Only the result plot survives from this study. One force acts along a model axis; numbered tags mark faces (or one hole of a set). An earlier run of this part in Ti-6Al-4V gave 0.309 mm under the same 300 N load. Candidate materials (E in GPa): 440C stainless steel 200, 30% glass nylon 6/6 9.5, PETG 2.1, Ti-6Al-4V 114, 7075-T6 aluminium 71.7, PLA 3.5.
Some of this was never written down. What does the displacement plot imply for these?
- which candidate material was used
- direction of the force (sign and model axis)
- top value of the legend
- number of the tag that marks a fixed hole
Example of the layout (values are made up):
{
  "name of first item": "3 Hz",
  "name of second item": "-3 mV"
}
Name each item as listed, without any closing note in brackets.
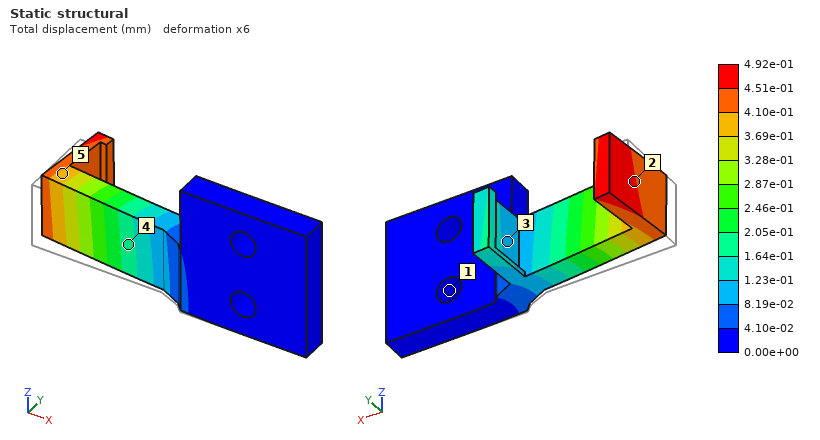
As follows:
{
  "which candidate material was used": "7075-T6 aluminium",
  "direction of the force": "+Y",
  "top value of the legend": "4.92e-01 mm",
  "number of the tag that marks a fixed hole": "1"
}
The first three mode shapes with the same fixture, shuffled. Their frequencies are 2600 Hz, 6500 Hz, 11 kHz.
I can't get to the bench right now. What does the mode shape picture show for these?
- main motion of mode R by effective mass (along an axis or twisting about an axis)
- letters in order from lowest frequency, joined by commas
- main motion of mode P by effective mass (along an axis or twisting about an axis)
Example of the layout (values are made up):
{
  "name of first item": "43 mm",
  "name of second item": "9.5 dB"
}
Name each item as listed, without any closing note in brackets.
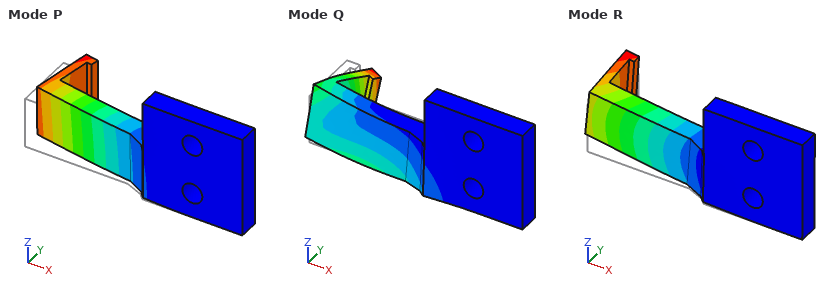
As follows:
{
  "main motion of mode R by effective mass": "along Z",
  "letters in order from lowest frequency, joined by commas": "P, R, Q",
  "main motion of mode P by effective mass": "along Y"
}
